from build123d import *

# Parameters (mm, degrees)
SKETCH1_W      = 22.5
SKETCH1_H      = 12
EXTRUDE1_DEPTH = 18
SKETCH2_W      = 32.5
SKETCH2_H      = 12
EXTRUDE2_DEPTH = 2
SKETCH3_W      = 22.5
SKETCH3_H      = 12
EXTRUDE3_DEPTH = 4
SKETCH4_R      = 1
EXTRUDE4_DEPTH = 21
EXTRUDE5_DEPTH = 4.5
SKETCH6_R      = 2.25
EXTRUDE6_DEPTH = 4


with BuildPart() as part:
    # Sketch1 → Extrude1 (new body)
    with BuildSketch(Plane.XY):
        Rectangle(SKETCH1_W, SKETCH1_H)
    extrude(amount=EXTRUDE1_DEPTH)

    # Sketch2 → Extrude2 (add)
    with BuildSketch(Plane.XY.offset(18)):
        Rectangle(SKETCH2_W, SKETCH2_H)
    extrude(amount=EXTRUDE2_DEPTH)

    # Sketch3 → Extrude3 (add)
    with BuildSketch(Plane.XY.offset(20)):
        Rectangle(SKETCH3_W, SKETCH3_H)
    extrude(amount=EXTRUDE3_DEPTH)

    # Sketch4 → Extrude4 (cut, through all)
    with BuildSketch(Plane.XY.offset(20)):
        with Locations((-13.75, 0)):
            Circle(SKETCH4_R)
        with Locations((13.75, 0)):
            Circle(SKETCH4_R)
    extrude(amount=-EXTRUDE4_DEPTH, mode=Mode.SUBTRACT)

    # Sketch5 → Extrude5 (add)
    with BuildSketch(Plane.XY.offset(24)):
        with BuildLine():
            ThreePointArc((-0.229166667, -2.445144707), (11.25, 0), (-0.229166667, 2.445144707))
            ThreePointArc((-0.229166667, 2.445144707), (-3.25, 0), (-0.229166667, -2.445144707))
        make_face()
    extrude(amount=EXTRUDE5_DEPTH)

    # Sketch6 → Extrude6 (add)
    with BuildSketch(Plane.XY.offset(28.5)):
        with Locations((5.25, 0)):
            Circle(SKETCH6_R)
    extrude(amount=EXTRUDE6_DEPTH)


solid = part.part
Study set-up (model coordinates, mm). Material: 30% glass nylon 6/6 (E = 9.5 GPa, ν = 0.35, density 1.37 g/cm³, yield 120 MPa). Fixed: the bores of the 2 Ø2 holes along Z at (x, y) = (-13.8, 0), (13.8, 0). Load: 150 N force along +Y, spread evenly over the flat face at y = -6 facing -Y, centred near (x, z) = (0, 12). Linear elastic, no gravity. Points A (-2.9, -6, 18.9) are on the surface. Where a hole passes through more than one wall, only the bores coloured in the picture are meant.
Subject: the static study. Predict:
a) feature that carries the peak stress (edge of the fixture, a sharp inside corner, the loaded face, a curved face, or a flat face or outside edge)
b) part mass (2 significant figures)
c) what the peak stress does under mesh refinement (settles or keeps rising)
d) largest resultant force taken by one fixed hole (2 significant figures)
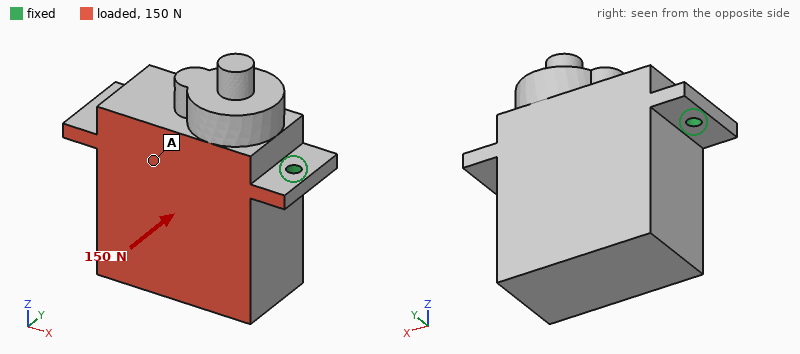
edge of the fixture
10 g
keeps rising
75 N
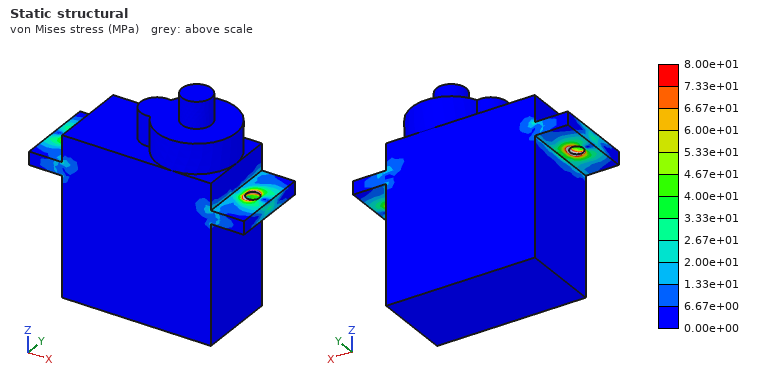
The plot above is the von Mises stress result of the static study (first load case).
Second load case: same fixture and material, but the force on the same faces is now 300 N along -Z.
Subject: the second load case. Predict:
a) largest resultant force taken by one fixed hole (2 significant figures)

150 N
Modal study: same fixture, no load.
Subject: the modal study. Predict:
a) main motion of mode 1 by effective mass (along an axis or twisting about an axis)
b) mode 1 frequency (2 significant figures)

along Y
1400 Hz
